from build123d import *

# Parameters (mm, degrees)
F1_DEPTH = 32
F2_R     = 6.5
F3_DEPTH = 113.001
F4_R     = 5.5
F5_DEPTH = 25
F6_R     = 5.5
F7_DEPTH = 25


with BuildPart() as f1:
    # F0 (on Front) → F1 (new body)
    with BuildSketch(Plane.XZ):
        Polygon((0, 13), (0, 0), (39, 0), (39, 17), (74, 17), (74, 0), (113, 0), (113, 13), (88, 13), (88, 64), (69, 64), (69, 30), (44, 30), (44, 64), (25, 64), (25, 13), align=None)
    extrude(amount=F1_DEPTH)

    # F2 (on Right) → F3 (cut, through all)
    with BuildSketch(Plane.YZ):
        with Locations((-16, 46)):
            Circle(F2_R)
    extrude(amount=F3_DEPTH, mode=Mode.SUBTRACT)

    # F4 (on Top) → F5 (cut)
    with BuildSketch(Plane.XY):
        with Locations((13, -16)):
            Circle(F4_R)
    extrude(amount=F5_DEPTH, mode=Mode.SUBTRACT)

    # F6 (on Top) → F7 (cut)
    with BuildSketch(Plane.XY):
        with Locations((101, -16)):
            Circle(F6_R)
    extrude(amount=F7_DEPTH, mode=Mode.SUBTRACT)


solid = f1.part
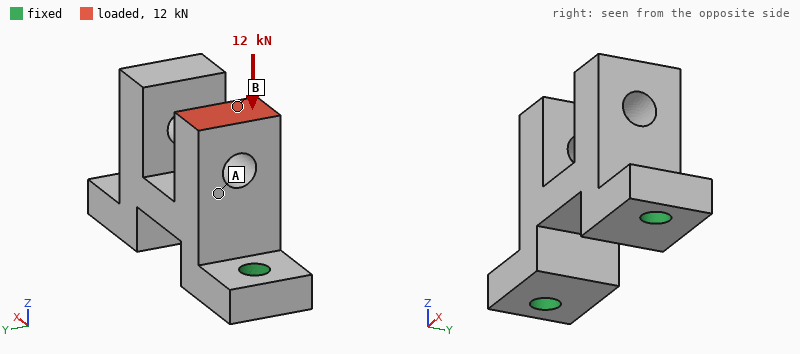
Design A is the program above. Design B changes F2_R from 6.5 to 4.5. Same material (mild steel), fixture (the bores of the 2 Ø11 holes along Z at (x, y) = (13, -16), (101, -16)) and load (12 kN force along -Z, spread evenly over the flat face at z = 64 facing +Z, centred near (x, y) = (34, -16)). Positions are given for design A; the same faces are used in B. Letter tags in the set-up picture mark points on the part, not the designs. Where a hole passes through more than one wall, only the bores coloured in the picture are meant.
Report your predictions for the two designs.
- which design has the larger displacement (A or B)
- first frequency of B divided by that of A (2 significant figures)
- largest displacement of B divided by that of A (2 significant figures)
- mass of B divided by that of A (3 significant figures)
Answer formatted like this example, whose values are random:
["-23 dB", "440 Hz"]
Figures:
["A", "0.98", "0.92", "1.03"]
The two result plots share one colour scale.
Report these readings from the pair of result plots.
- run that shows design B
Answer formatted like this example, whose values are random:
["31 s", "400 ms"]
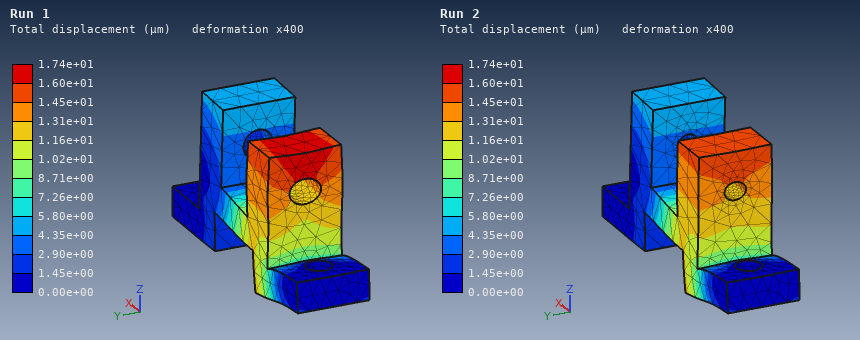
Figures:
["Run 2"]
